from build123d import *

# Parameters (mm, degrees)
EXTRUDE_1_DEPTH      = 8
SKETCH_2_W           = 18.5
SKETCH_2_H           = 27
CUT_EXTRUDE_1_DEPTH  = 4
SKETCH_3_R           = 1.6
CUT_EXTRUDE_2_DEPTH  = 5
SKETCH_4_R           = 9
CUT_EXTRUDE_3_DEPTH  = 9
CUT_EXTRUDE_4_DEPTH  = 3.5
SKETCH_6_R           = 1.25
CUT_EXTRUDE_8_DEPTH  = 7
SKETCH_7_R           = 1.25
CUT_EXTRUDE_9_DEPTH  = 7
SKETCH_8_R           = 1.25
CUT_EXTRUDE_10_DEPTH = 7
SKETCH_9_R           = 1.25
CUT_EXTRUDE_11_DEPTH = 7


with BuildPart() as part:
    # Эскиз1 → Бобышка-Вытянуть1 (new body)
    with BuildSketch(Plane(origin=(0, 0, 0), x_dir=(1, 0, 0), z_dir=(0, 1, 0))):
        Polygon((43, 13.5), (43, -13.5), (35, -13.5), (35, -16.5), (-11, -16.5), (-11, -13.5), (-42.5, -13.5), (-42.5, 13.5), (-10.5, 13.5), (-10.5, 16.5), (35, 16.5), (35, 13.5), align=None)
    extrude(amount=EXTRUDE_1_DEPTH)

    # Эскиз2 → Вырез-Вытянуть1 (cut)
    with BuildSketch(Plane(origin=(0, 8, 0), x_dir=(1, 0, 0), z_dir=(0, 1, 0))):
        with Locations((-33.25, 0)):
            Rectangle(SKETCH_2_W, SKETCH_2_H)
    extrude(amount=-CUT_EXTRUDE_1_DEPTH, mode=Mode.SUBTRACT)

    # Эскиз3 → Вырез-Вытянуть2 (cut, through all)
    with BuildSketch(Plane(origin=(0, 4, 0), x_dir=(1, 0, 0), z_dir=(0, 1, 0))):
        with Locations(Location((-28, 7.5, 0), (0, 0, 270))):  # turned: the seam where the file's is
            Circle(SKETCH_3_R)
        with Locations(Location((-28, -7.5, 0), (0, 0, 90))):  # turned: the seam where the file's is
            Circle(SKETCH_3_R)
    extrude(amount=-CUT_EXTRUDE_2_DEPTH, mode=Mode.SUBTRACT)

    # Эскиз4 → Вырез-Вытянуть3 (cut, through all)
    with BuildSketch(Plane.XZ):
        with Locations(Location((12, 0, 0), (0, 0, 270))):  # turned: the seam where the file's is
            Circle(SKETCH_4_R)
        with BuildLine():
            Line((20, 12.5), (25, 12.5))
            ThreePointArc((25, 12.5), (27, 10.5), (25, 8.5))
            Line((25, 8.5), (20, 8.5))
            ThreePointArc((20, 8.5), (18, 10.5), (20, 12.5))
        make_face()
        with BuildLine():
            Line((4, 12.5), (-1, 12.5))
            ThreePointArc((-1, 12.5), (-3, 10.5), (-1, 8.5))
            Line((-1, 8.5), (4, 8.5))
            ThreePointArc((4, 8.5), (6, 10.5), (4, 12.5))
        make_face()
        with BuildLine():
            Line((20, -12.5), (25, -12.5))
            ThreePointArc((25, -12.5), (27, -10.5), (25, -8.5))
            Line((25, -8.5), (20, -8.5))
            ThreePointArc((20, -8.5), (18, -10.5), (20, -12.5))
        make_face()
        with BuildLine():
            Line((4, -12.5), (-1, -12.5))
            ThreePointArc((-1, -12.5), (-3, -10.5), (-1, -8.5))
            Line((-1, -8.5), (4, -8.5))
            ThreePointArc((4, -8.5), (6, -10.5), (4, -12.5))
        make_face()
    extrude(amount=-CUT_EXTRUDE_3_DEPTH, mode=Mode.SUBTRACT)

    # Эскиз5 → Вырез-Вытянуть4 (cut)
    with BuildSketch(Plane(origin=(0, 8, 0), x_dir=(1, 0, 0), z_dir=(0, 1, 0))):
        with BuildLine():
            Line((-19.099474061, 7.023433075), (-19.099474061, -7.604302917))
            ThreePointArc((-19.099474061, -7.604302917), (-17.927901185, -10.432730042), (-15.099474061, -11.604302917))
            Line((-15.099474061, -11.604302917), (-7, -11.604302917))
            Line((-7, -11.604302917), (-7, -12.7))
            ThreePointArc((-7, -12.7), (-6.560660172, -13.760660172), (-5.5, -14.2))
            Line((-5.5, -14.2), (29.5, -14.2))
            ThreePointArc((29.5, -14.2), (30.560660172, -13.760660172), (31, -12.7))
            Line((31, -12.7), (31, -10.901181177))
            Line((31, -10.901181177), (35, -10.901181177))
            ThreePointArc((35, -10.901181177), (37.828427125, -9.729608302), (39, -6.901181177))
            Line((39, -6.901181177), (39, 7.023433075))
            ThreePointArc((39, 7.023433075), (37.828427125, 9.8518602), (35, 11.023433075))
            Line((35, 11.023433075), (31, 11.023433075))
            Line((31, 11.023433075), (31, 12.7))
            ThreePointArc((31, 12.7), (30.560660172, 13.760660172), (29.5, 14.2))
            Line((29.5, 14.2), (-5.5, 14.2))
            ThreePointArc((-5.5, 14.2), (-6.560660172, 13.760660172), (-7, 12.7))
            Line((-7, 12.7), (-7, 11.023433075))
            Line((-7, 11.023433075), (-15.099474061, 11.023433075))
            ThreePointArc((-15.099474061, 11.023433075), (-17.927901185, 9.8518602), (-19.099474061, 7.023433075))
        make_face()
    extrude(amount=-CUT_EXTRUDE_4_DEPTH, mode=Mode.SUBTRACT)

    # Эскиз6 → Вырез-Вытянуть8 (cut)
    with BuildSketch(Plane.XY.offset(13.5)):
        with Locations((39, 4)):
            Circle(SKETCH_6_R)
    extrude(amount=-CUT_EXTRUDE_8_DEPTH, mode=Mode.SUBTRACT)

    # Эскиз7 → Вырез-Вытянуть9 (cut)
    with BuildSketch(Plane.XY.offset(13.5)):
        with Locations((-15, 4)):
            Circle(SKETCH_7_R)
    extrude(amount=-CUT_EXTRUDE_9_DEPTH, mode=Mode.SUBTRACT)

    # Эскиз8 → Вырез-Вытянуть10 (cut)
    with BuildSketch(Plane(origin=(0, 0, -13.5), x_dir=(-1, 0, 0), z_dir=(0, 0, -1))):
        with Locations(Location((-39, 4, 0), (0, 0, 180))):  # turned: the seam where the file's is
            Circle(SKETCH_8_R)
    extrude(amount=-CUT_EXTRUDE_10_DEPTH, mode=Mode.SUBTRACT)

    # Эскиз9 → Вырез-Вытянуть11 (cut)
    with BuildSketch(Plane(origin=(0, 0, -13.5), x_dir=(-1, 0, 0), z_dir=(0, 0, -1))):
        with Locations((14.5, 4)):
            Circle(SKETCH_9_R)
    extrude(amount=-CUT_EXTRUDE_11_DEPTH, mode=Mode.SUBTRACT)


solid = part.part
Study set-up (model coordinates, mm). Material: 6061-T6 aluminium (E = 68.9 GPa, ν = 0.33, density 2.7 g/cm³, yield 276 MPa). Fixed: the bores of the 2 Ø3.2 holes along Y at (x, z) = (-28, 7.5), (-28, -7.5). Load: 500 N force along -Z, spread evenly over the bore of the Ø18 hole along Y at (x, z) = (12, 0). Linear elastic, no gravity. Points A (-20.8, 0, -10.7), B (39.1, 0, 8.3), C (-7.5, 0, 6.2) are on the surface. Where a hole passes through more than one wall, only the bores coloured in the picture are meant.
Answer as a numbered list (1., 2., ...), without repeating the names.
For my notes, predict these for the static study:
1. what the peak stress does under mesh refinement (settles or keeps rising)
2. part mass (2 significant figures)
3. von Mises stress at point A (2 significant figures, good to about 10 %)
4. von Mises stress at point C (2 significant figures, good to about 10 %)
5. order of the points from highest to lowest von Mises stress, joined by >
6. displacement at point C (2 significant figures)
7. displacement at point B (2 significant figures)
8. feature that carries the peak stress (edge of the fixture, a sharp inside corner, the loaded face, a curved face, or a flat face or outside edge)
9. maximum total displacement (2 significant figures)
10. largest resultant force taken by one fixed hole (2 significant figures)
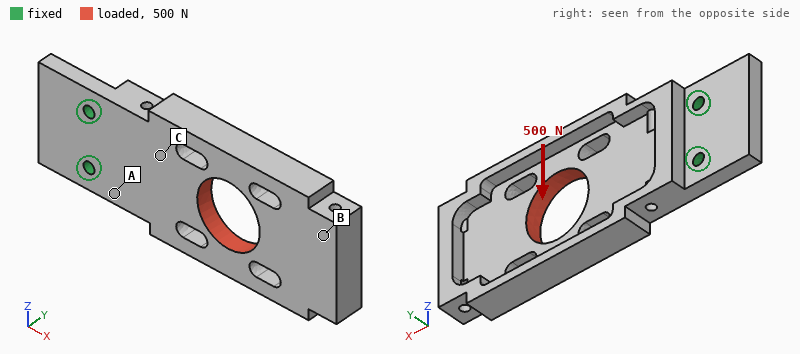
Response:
1. keeps rising
2. 31 g
3. 27 MPa
4. 12 MPa
5. A > C > B
6. 15 µm
7. 63 µm
8. edge of the fixture
9. 70 µm
10. 1.2 kN
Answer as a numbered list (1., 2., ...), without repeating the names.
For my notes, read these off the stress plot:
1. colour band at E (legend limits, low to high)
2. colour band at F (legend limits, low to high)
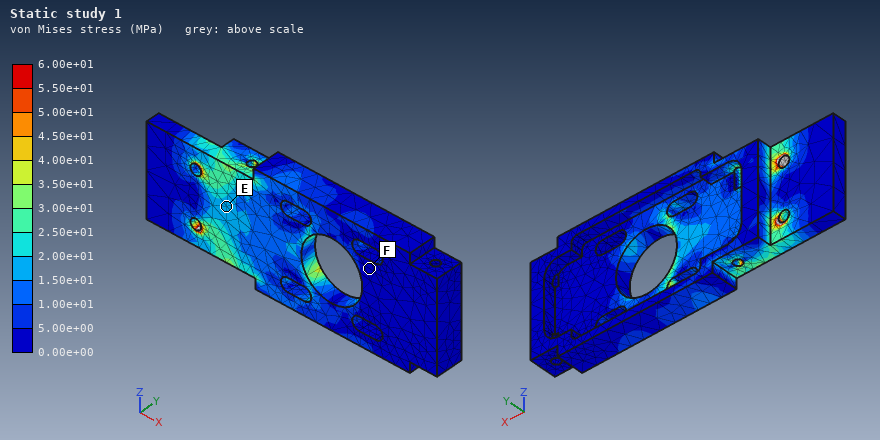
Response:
1. 1.50e+01 to 2.00e+01 MPa
2. 0.00e+00 to 5.00e+00 MPa
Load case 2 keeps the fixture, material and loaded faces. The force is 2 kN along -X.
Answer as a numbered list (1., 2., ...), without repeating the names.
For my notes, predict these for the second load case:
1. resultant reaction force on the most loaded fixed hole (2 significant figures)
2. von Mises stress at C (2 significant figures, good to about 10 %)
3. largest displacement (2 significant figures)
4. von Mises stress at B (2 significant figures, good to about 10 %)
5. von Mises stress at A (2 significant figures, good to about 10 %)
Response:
1. 1.0 kN
2. 20 MPa
3. 52 µm
4. 5.4 MPa
5. 22 MPa
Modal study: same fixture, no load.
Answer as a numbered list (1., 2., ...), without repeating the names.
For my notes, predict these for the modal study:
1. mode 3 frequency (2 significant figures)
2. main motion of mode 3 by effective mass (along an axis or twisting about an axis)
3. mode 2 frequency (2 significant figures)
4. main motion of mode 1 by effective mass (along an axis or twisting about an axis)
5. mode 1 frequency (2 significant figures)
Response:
1. 3200 Hz
2. along Z
3. 2600 Hz
4. along Y
5. 750 Hz
